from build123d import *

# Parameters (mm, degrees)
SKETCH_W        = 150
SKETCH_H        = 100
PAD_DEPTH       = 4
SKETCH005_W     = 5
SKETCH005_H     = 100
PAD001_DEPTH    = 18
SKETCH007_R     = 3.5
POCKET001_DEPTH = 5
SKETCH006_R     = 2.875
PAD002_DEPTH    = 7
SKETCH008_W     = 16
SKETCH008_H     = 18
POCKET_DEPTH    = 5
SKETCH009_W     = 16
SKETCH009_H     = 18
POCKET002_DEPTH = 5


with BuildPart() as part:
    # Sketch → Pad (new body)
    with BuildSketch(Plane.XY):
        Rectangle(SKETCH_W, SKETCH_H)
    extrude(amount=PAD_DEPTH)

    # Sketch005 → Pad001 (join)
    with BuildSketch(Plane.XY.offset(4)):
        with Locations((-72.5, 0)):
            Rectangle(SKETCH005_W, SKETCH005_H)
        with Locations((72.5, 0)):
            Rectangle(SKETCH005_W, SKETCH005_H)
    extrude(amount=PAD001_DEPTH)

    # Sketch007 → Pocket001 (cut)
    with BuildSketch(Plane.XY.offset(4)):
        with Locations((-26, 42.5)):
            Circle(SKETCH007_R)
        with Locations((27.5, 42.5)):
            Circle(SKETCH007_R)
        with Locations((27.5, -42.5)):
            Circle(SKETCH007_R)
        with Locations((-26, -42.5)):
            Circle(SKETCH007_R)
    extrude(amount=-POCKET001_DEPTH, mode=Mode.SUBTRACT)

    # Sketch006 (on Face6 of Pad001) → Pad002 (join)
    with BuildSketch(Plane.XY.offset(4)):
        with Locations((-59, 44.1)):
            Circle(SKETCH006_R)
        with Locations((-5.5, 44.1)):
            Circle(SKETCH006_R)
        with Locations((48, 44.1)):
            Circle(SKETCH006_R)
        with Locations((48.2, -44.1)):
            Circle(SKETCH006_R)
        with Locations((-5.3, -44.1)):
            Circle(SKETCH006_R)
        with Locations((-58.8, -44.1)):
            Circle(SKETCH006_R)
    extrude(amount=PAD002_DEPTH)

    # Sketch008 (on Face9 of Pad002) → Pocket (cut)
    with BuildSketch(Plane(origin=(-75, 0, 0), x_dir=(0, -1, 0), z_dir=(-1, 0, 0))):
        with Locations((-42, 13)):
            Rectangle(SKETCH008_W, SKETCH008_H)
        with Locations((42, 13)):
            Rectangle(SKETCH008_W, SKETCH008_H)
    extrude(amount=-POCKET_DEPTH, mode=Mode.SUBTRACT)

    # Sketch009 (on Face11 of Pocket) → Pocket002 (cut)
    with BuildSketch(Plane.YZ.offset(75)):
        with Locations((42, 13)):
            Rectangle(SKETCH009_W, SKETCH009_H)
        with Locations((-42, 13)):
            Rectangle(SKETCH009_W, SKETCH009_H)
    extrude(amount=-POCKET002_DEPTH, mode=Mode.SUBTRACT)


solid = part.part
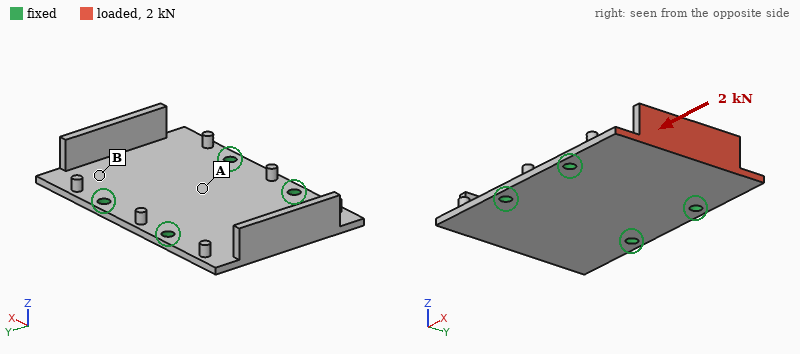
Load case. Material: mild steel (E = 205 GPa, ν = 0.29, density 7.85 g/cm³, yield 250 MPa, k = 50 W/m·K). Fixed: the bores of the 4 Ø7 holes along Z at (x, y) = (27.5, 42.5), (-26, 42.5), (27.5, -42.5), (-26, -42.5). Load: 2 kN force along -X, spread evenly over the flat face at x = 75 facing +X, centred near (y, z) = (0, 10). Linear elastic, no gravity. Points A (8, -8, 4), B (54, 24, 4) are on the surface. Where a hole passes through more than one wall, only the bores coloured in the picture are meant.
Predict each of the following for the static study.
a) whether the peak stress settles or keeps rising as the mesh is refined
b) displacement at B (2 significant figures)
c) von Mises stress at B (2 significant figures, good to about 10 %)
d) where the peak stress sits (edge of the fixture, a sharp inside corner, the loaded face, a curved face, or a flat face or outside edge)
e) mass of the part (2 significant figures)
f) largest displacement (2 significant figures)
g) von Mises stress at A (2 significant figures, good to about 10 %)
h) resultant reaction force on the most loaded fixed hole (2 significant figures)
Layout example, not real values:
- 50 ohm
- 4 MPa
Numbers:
- keeps rising
- 0.066 mm
- 62 MPa
- edge of the fixture
- 570 g
- 0.24 mm
- 14 MPa
- 730 N
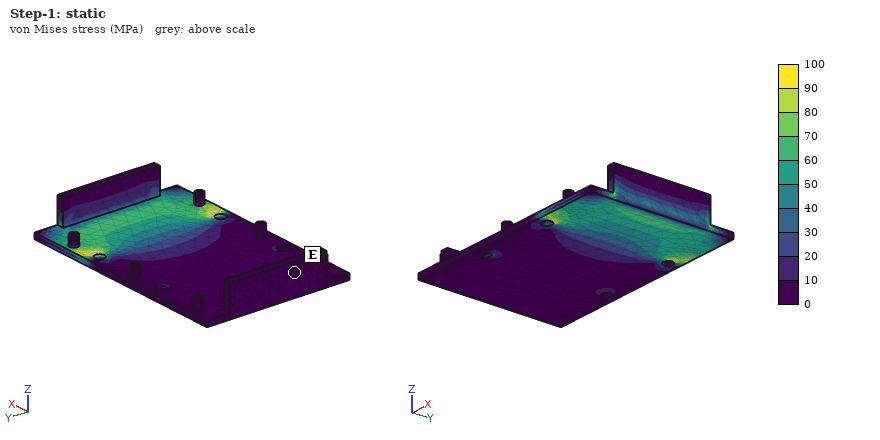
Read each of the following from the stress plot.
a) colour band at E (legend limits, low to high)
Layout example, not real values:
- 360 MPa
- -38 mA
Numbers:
- 0 to 10 MPa
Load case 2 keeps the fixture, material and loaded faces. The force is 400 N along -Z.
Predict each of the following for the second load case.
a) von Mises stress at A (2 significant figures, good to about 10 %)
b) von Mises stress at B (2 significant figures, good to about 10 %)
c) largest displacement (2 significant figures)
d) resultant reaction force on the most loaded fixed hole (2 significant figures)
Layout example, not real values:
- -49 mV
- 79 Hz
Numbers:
- 14 MPa
- 31 MPa
- 0.18 mm
- 260 N
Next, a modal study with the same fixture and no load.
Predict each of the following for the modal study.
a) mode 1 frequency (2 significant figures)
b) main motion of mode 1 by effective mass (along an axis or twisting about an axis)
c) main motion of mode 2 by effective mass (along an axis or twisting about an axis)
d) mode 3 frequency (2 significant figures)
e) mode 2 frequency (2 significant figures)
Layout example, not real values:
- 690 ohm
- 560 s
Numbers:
- 820 Hz
- along Z
- along Z
- 1800 Hz
- 860 Hz
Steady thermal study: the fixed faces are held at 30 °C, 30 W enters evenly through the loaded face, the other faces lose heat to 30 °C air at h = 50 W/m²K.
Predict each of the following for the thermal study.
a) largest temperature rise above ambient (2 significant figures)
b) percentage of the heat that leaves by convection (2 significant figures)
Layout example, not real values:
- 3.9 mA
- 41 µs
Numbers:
- 60 K
- 62 %
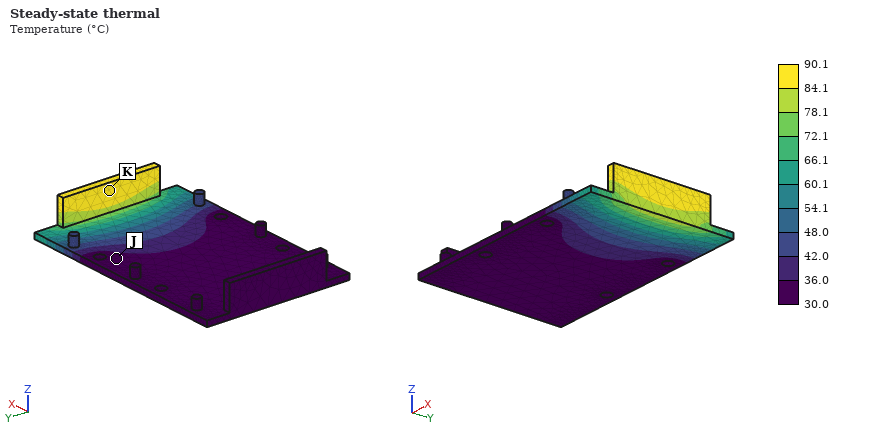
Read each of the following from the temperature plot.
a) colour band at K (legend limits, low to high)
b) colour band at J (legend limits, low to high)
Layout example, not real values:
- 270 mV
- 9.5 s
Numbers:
- 84.1 to 90.1 °C
- 30.0 to 36.0 °C
